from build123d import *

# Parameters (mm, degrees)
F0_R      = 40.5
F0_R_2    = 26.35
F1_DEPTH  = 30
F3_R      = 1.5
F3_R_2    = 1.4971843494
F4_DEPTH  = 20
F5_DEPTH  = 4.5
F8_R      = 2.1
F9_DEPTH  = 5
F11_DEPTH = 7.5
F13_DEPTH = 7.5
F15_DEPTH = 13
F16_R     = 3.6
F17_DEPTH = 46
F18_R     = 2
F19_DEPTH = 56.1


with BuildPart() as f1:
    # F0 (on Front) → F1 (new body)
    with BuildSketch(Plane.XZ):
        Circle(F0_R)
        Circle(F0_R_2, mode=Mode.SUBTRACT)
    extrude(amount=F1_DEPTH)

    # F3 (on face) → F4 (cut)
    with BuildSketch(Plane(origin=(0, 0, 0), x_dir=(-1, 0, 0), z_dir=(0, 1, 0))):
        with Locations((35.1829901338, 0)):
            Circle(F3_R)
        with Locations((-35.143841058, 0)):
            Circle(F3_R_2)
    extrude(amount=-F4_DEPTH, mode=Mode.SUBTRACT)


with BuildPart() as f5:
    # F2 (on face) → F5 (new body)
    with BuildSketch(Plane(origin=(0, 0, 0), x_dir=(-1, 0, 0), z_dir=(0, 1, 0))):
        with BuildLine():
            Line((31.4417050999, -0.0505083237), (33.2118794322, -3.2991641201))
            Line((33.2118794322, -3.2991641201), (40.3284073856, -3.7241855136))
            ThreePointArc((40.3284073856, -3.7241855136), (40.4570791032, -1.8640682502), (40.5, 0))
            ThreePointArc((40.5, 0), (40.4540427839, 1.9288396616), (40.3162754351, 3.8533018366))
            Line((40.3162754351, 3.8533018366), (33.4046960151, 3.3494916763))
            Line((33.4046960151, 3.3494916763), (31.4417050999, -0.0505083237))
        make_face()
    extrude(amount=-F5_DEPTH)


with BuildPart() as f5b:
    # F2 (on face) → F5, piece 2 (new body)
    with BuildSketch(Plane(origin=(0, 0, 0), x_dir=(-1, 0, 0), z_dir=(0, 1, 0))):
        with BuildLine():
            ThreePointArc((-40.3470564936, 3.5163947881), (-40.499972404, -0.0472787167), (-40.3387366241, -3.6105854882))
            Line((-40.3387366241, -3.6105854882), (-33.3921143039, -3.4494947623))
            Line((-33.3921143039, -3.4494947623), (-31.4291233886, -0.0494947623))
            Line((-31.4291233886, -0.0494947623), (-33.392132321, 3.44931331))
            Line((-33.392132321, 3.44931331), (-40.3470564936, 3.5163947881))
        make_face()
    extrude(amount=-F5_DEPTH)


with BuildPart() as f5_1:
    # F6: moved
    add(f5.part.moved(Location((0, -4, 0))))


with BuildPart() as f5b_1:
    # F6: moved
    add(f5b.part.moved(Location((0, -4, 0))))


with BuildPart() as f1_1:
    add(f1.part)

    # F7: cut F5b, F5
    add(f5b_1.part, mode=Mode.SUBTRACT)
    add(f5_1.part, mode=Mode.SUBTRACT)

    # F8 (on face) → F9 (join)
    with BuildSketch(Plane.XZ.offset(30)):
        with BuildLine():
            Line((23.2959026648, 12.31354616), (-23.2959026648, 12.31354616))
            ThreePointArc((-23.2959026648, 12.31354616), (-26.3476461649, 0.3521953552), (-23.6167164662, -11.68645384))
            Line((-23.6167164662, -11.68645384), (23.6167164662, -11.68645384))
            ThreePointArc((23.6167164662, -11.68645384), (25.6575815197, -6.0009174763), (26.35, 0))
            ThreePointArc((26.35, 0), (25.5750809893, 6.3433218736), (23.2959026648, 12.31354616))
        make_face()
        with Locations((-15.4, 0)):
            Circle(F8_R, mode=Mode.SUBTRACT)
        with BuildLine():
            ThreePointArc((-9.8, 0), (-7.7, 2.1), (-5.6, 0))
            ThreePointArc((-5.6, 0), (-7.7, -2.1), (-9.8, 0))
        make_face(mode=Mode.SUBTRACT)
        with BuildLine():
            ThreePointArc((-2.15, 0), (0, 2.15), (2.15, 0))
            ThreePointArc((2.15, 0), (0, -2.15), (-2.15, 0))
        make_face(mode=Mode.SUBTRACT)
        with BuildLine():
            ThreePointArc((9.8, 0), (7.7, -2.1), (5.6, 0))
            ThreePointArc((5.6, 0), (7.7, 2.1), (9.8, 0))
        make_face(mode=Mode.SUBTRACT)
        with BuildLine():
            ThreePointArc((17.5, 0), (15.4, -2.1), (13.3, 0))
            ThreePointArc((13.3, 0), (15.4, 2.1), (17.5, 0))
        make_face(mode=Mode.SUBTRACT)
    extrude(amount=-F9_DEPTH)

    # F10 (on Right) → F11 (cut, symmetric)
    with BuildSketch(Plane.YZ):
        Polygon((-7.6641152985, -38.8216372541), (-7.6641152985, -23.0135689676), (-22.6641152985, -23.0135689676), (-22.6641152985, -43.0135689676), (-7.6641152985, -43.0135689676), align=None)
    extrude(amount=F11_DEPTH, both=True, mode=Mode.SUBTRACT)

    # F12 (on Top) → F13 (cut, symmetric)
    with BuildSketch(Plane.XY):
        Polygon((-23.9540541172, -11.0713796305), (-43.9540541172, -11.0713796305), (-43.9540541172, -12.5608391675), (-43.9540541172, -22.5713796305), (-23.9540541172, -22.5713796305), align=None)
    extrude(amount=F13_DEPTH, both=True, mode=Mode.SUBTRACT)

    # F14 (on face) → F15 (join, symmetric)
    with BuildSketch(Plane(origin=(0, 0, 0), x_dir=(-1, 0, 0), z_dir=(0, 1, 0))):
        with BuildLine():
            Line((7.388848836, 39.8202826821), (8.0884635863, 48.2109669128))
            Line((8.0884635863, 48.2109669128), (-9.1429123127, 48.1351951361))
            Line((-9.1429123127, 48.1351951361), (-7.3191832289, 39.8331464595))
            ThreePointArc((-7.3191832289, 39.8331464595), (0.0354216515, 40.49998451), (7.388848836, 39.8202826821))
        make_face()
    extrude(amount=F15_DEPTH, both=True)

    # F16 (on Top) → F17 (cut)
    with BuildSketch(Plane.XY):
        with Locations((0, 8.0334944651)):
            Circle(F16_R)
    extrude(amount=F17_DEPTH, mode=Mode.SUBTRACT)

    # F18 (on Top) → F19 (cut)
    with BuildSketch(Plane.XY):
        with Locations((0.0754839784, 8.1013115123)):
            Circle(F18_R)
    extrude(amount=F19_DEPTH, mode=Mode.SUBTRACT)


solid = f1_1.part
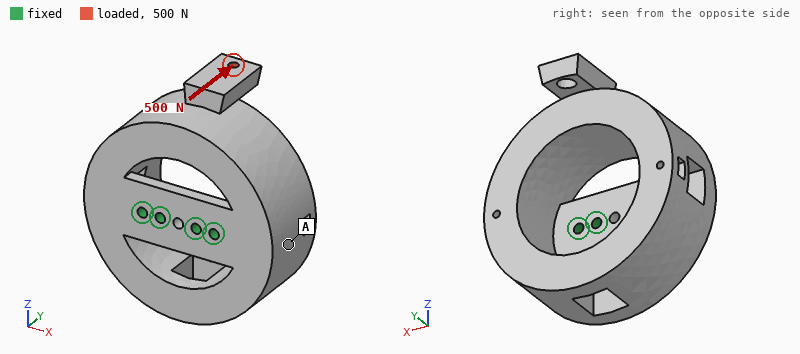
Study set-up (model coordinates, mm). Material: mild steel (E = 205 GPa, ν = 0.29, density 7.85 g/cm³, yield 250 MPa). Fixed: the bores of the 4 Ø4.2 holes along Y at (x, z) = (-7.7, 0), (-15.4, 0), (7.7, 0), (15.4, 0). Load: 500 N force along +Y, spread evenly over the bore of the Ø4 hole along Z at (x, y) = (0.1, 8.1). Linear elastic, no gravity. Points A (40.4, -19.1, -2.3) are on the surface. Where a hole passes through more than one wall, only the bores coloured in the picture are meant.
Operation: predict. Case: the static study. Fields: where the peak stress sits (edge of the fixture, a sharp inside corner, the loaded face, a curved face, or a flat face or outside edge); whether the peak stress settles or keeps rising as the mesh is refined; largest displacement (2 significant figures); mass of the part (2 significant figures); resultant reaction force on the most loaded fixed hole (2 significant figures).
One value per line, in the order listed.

edge of the fixture
keeps rising
91 µm
720 g
270 N
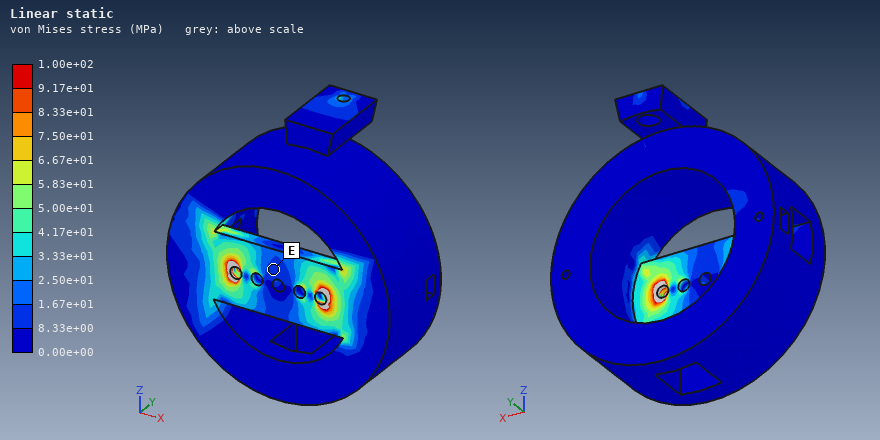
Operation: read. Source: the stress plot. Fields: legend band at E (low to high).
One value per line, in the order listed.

8.33e+00 to 1.67e+01 MPa
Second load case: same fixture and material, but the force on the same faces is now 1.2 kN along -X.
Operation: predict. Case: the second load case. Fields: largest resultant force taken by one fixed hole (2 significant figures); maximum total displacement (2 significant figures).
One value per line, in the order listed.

2.0 kN
33 µm
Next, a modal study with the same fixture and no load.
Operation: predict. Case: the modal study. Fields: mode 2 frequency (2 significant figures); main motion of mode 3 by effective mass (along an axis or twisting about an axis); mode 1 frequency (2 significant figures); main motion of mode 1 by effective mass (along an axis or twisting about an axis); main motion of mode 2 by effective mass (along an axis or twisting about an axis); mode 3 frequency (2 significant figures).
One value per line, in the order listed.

2500 Hz
twisting about Y
860 Hz
along Z
along X
3100 Hz
